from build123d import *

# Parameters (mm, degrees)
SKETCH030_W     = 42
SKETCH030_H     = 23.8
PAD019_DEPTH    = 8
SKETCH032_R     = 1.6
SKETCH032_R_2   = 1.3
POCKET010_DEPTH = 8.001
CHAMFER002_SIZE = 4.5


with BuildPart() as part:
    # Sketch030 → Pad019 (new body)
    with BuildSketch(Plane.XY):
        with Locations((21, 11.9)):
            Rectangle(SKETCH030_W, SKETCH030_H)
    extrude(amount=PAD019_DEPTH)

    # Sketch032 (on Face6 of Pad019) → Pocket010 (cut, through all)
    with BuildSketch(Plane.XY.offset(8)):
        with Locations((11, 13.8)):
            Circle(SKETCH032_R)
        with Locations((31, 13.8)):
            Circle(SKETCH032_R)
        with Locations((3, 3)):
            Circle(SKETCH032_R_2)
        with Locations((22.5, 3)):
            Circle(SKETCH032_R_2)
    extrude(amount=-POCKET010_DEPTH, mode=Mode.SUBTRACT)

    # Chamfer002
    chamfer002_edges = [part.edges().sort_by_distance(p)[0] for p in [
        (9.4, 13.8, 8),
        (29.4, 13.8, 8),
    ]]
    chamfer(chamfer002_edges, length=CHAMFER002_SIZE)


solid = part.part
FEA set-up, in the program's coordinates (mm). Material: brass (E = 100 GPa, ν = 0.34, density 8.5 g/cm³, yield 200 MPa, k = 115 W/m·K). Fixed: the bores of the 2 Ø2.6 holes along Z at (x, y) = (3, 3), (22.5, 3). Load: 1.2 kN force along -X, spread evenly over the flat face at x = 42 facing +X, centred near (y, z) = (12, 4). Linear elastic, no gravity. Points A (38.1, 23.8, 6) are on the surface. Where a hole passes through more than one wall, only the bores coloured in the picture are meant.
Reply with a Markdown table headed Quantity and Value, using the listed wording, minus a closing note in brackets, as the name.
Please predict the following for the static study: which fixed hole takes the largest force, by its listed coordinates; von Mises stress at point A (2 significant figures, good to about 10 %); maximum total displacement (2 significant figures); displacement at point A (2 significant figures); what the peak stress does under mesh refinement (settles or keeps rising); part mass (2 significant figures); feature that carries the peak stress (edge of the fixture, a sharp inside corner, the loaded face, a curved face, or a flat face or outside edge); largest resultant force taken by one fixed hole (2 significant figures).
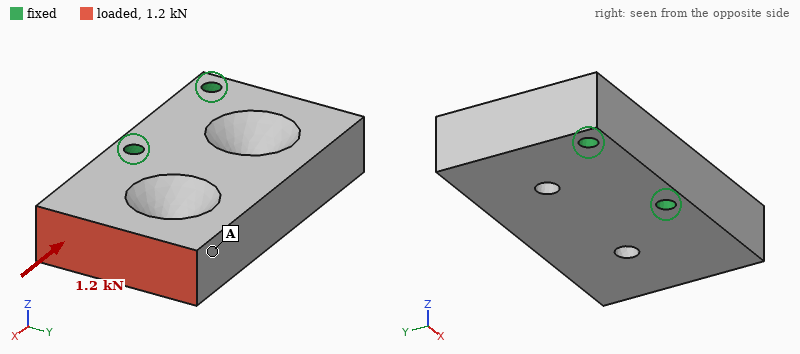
| Quantity | Value |
|---|---|
| which fixed hole takes the largest force, by its listed coordinates | (22.5, 3) |
| von Mises stress at point A | 7.1 MPa |
| maximum total displacement | 7.3 µm |
| displacement at point A | 6.5 µm |
| what the peak stress does under mesh refinement | keeps rising |
| part mass | 63 g |
| feature that carries the peak stress | edge of the fixture |
| largest resultant force taken by one fixed hole | 950 N |
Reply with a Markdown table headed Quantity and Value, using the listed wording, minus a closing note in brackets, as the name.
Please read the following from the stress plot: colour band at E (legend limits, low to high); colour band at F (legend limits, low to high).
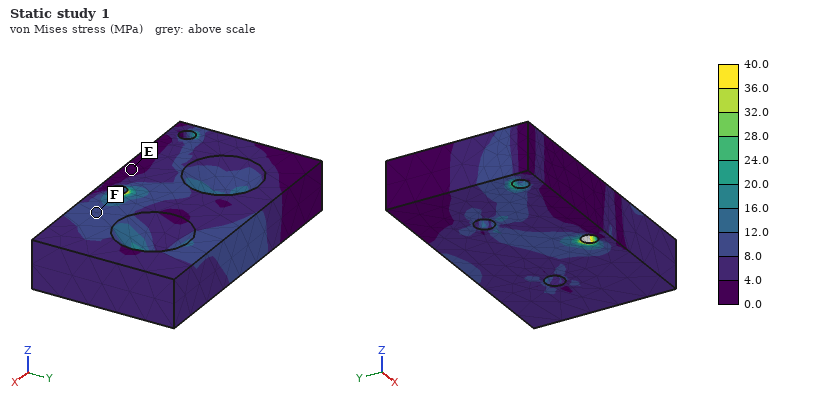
| Quantity | Value |
|---|---|
| colour band at E | 0.0 to 4.0 MPa |
| colour band at F | 8.0 to 12.0 MPa |
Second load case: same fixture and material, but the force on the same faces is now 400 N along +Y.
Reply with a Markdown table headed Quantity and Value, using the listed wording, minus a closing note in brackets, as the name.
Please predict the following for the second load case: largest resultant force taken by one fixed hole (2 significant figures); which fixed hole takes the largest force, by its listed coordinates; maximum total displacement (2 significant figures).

| Quantity | Value |
|---|---|
| largest resultant force taken by one fixed hole | 770 N |
| which fixed hole takes the largest force, by its listed coordinates | (22.5, 3) |
| maximum total displacement | 7.6 µm |
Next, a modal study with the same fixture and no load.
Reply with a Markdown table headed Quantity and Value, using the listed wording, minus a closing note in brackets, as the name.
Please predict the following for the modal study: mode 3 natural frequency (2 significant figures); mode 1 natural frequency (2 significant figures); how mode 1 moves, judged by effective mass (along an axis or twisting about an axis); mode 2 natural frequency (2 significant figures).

| Quantity | Value |
|---|---|
| mode 3 natural frequency | 9800 Hz |
| mode 1 natural frequency | 5700 Hz |
| how mode 1 moves, judged by effective mass | along Z |
| mode 2 natural frequency | 8400 Hz |
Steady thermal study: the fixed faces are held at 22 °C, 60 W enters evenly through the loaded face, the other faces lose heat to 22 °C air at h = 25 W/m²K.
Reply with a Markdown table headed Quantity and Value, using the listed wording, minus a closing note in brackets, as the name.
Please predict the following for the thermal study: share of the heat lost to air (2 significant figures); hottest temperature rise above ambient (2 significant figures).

| Quantity | Value |
|---|---|
| share of the heat lost to air | 3.2 % |
| hottest temperature rise above ambient | 78 K |
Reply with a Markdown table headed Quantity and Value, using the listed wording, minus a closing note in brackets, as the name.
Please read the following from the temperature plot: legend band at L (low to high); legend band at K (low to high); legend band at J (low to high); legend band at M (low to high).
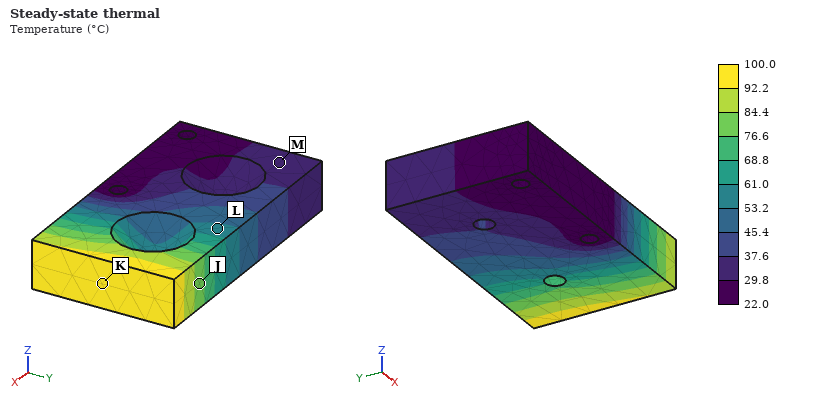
| Quantity | Value |
|---|---|
| legend band at L | 53.2 to 61.0 °C |
| legend band at K | 92.2 to 100.0 °C |
| legend band at J | 76.6 to 84.4 °C |
| legend band at M | 29.8 to 37.6 °C |
